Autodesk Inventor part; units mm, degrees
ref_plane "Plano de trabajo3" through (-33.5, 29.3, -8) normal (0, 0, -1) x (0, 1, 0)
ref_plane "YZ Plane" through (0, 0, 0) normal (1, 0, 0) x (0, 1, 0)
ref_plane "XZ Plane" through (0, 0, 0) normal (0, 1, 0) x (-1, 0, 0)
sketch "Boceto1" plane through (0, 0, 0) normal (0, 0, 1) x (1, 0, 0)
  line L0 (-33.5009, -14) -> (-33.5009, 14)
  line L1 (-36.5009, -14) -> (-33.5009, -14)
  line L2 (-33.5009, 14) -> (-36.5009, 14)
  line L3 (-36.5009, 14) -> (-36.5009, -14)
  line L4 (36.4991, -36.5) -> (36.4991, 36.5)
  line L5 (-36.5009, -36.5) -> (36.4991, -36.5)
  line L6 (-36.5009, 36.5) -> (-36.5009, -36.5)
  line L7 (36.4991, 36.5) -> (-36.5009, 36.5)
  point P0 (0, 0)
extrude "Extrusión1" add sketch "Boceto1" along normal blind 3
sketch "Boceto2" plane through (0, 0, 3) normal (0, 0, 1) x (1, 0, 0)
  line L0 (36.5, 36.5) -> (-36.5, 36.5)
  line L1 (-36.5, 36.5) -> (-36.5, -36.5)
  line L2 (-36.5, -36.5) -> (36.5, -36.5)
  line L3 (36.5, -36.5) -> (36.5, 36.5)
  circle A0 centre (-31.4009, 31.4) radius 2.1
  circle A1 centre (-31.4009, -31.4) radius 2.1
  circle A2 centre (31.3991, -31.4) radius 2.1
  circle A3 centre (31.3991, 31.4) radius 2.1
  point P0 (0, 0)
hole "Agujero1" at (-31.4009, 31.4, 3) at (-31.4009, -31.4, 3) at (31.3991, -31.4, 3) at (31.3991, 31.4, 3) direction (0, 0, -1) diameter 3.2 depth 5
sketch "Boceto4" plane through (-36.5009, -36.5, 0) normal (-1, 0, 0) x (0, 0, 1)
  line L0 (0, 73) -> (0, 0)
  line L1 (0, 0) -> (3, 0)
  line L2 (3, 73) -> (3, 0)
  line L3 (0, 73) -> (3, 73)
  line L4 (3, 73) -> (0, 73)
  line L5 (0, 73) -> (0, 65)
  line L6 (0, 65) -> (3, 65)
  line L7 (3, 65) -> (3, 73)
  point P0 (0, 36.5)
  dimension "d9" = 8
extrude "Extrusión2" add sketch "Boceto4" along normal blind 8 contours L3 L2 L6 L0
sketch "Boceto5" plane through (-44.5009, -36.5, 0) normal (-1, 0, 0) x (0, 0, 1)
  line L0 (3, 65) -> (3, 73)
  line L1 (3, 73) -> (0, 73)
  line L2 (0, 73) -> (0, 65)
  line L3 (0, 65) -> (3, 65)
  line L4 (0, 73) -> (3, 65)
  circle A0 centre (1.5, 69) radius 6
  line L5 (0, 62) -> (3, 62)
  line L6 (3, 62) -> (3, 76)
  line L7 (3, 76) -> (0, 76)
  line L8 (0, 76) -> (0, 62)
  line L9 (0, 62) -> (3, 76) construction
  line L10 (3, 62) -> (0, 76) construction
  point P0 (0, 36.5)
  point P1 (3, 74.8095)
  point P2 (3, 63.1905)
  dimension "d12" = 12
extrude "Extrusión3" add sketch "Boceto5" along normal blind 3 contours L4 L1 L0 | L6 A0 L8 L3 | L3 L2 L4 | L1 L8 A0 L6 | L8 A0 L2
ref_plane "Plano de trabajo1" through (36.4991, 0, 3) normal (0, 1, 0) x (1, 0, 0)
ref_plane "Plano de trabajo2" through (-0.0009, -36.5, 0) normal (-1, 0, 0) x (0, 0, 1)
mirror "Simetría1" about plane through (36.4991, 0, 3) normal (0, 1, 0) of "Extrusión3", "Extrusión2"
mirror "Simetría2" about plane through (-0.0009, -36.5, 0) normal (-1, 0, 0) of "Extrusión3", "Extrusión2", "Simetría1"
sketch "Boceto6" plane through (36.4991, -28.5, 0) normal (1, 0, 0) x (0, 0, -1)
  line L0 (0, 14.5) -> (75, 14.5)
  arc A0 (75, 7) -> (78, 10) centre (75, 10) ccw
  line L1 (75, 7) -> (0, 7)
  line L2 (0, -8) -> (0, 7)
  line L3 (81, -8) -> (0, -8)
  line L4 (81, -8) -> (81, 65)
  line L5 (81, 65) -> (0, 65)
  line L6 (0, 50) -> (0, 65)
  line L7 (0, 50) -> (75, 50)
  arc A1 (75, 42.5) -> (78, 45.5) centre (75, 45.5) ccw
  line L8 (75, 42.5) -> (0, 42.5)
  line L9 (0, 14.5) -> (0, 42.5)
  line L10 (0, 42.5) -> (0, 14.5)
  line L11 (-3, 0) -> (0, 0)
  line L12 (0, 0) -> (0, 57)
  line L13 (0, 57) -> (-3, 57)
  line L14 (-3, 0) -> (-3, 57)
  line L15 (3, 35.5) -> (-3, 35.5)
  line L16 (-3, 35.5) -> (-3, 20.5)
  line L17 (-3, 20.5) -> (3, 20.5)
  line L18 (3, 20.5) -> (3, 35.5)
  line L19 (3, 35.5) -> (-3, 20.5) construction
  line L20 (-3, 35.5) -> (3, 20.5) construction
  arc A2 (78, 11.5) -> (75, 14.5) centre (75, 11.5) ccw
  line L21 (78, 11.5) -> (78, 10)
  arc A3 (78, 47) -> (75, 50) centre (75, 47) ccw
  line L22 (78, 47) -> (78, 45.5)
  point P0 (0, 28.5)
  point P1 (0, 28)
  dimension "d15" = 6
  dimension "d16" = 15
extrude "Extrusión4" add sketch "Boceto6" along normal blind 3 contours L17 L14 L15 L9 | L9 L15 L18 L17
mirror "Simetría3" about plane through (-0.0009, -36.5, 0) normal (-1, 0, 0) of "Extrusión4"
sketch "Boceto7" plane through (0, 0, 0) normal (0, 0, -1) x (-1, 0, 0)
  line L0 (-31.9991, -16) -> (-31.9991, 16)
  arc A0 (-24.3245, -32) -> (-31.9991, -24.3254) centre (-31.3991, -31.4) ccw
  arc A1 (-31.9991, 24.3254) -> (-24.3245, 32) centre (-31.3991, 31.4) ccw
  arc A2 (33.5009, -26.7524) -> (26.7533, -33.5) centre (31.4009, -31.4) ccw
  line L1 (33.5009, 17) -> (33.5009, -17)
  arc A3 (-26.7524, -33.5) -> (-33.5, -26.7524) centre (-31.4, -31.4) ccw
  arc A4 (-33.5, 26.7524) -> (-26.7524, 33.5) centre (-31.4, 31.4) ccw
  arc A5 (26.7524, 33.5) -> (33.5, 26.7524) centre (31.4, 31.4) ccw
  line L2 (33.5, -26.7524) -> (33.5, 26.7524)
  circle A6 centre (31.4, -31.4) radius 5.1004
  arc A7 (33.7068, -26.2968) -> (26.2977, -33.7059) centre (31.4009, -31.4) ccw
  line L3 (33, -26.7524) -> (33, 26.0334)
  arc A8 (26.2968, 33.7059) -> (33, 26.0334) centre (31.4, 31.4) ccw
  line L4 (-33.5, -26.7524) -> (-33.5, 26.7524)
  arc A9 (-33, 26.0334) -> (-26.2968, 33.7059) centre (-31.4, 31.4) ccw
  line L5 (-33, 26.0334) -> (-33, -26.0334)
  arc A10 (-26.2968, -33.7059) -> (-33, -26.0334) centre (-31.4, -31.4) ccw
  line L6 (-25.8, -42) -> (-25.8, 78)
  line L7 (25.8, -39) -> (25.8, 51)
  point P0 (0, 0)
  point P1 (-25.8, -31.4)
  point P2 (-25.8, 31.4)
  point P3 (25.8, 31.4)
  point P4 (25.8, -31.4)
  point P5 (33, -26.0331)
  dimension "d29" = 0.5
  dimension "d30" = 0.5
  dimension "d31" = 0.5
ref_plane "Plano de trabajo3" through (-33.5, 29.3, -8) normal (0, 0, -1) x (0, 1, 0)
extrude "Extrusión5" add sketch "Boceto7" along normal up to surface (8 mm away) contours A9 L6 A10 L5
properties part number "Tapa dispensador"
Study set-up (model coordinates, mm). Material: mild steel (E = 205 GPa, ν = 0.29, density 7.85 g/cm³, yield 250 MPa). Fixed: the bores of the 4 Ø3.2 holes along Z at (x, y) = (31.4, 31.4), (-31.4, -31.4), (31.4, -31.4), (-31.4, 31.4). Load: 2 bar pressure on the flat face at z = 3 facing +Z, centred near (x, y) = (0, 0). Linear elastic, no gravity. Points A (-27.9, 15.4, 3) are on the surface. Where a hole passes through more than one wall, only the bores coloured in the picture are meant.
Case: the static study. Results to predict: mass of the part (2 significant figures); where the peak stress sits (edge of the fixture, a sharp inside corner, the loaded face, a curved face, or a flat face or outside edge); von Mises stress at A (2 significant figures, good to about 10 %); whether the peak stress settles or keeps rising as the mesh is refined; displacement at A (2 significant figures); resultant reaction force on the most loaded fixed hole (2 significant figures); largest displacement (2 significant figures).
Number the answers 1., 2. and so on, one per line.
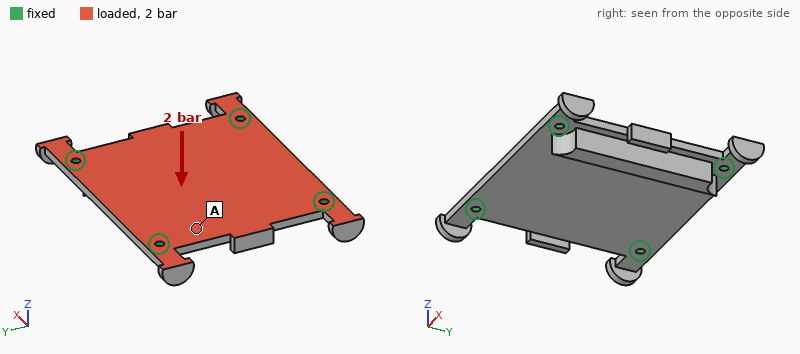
1. 170 g
2. edge of the fixture
3. 16 MPa
4. keeps rising
5. 18 µm
6. 360 N
7. 38 µm
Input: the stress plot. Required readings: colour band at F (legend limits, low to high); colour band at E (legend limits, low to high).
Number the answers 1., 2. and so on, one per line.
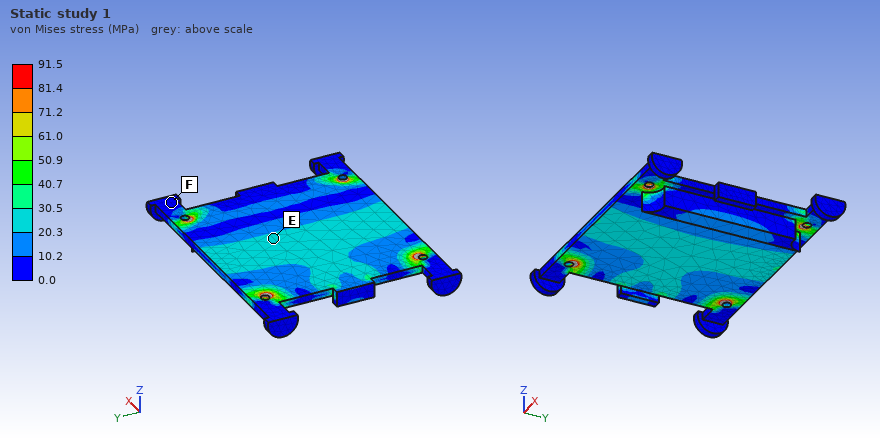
1. 0.0 to 10.2 MPa
2. 20.3 to 30.5 MPa
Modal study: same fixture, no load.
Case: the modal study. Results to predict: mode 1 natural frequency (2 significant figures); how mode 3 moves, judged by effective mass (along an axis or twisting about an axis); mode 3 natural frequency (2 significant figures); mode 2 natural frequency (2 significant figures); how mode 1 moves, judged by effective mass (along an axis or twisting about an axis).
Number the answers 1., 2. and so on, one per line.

1. 2800 Hz
2. twisting about X
3. 4600 Hz
4. 4200 Hz
5. along Z
